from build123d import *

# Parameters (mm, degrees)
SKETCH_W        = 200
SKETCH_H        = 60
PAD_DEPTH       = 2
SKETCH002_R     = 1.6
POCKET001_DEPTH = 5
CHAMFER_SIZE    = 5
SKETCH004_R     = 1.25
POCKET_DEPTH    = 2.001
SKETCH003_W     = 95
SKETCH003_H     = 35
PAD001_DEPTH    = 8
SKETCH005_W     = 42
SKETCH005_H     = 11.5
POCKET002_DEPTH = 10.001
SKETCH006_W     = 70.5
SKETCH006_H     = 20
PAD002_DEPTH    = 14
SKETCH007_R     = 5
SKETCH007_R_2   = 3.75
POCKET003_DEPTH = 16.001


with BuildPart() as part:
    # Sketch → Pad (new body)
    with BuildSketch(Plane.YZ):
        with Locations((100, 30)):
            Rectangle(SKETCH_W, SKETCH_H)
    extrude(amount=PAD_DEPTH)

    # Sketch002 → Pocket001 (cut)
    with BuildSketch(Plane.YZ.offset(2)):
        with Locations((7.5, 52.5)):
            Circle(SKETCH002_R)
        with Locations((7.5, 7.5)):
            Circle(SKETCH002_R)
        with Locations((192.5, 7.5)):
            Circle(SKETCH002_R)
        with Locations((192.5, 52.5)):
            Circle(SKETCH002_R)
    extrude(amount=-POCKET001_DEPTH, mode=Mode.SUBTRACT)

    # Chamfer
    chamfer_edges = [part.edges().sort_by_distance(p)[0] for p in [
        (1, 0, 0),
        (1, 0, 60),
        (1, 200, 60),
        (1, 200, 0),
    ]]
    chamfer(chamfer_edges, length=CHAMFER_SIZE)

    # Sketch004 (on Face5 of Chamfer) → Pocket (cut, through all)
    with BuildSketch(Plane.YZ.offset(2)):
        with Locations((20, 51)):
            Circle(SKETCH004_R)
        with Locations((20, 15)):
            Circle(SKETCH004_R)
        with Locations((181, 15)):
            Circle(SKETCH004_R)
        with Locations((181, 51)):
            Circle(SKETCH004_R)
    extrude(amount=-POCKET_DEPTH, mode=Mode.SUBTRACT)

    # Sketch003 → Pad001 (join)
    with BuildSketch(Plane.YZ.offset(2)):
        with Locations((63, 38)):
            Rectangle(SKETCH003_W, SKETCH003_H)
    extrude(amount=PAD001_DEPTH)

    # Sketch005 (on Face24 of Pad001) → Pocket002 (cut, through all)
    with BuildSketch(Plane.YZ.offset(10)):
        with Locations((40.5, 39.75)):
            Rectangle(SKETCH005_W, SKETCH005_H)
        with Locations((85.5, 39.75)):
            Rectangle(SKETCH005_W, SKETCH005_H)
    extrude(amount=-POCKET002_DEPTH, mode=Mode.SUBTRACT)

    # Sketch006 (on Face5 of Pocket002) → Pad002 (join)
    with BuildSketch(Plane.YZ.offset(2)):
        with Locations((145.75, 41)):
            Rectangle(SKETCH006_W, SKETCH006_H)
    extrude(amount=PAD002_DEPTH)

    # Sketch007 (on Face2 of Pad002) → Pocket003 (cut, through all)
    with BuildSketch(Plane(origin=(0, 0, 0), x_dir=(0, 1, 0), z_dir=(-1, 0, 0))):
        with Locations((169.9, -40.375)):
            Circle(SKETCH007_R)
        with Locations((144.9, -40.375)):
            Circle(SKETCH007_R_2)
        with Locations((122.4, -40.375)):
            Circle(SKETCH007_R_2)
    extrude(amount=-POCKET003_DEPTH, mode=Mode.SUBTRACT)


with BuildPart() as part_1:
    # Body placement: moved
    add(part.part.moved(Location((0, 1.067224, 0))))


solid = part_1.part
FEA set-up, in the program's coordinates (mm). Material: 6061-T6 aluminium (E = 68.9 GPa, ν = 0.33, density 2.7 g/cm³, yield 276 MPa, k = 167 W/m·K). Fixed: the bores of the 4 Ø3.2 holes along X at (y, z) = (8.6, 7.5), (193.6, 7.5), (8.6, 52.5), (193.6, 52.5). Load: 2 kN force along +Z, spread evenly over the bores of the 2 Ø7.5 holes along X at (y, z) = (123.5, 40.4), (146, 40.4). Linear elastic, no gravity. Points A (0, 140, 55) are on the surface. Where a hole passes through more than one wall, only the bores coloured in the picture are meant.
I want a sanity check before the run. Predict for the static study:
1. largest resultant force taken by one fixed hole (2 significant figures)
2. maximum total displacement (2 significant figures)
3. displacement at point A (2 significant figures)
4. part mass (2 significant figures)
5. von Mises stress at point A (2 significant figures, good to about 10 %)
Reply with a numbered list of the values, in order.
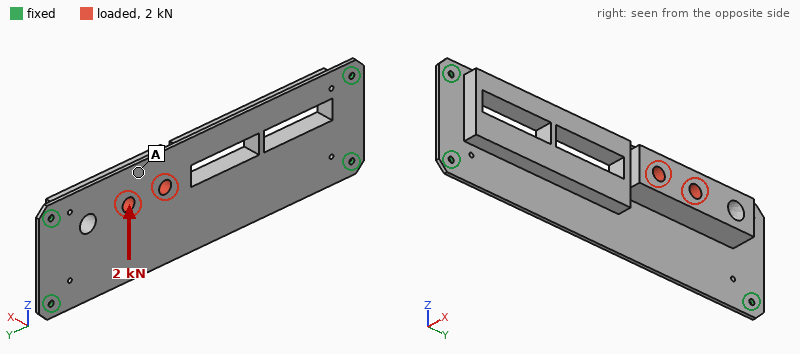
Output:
1. 1.3 kN
2. 0.30 mm
3. 0.12 mm
4. 160 g
5. 14 MPa
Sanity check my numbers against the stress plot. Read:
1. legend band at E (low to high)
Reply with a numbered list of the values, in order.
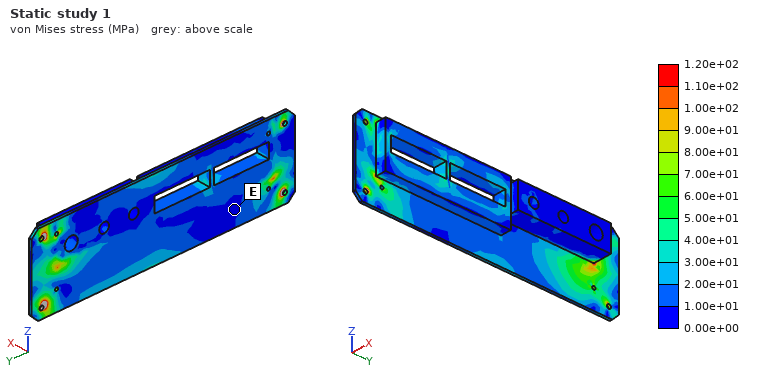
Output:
1. 0.00e+00 to 1.00e+01 MPa
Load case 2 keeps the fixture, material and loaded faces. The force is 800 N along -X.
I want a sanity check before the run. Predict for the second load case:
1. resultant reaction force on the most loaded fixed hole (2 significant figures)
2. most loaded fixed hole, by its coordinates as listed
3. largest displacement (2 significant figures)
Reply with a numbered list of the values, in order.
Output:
1. 1.2 kN
2. (193.6, 52.5)
3. 0.38 mm
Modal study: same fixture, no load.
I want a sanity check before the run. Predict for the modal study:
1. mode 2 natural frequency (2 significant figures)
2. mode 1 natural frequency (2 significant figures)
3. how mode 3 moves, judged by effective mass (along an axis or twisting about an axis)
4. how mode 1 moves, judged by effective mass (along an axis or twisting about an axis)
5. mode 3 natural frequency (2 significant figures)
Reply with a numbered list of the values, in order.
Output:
1. 1400 Hz
2. 750 Hz
3. twisting about Z
4. along X
5. 2000 Hz
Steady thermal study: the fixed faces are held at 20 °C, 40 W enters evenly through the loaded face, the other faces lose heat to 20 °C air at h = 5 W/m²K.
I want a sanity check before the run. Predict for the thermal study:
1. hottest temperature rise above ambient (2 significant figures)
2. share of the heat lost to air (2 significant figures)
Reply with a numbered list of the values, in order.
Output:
1. 47 K
2. 10 %
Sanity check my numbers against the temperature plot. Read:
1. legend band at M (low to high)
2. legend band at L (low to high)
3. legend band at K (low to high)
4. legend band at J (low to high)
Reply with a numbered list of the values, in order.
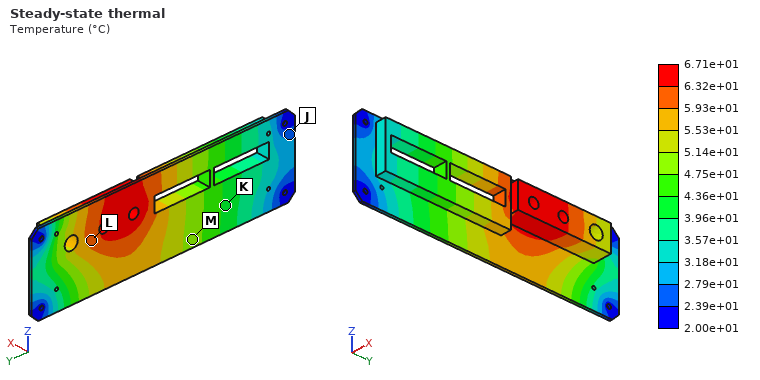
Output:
1. 4.75e+01 to 5.14e+01 °C
2. 5.93e+01 to 6.32e+01 °C
3. 3.96e+01 to 4.36e+01 °C
4. 2.39e+01 to 2.79e+01 °C
